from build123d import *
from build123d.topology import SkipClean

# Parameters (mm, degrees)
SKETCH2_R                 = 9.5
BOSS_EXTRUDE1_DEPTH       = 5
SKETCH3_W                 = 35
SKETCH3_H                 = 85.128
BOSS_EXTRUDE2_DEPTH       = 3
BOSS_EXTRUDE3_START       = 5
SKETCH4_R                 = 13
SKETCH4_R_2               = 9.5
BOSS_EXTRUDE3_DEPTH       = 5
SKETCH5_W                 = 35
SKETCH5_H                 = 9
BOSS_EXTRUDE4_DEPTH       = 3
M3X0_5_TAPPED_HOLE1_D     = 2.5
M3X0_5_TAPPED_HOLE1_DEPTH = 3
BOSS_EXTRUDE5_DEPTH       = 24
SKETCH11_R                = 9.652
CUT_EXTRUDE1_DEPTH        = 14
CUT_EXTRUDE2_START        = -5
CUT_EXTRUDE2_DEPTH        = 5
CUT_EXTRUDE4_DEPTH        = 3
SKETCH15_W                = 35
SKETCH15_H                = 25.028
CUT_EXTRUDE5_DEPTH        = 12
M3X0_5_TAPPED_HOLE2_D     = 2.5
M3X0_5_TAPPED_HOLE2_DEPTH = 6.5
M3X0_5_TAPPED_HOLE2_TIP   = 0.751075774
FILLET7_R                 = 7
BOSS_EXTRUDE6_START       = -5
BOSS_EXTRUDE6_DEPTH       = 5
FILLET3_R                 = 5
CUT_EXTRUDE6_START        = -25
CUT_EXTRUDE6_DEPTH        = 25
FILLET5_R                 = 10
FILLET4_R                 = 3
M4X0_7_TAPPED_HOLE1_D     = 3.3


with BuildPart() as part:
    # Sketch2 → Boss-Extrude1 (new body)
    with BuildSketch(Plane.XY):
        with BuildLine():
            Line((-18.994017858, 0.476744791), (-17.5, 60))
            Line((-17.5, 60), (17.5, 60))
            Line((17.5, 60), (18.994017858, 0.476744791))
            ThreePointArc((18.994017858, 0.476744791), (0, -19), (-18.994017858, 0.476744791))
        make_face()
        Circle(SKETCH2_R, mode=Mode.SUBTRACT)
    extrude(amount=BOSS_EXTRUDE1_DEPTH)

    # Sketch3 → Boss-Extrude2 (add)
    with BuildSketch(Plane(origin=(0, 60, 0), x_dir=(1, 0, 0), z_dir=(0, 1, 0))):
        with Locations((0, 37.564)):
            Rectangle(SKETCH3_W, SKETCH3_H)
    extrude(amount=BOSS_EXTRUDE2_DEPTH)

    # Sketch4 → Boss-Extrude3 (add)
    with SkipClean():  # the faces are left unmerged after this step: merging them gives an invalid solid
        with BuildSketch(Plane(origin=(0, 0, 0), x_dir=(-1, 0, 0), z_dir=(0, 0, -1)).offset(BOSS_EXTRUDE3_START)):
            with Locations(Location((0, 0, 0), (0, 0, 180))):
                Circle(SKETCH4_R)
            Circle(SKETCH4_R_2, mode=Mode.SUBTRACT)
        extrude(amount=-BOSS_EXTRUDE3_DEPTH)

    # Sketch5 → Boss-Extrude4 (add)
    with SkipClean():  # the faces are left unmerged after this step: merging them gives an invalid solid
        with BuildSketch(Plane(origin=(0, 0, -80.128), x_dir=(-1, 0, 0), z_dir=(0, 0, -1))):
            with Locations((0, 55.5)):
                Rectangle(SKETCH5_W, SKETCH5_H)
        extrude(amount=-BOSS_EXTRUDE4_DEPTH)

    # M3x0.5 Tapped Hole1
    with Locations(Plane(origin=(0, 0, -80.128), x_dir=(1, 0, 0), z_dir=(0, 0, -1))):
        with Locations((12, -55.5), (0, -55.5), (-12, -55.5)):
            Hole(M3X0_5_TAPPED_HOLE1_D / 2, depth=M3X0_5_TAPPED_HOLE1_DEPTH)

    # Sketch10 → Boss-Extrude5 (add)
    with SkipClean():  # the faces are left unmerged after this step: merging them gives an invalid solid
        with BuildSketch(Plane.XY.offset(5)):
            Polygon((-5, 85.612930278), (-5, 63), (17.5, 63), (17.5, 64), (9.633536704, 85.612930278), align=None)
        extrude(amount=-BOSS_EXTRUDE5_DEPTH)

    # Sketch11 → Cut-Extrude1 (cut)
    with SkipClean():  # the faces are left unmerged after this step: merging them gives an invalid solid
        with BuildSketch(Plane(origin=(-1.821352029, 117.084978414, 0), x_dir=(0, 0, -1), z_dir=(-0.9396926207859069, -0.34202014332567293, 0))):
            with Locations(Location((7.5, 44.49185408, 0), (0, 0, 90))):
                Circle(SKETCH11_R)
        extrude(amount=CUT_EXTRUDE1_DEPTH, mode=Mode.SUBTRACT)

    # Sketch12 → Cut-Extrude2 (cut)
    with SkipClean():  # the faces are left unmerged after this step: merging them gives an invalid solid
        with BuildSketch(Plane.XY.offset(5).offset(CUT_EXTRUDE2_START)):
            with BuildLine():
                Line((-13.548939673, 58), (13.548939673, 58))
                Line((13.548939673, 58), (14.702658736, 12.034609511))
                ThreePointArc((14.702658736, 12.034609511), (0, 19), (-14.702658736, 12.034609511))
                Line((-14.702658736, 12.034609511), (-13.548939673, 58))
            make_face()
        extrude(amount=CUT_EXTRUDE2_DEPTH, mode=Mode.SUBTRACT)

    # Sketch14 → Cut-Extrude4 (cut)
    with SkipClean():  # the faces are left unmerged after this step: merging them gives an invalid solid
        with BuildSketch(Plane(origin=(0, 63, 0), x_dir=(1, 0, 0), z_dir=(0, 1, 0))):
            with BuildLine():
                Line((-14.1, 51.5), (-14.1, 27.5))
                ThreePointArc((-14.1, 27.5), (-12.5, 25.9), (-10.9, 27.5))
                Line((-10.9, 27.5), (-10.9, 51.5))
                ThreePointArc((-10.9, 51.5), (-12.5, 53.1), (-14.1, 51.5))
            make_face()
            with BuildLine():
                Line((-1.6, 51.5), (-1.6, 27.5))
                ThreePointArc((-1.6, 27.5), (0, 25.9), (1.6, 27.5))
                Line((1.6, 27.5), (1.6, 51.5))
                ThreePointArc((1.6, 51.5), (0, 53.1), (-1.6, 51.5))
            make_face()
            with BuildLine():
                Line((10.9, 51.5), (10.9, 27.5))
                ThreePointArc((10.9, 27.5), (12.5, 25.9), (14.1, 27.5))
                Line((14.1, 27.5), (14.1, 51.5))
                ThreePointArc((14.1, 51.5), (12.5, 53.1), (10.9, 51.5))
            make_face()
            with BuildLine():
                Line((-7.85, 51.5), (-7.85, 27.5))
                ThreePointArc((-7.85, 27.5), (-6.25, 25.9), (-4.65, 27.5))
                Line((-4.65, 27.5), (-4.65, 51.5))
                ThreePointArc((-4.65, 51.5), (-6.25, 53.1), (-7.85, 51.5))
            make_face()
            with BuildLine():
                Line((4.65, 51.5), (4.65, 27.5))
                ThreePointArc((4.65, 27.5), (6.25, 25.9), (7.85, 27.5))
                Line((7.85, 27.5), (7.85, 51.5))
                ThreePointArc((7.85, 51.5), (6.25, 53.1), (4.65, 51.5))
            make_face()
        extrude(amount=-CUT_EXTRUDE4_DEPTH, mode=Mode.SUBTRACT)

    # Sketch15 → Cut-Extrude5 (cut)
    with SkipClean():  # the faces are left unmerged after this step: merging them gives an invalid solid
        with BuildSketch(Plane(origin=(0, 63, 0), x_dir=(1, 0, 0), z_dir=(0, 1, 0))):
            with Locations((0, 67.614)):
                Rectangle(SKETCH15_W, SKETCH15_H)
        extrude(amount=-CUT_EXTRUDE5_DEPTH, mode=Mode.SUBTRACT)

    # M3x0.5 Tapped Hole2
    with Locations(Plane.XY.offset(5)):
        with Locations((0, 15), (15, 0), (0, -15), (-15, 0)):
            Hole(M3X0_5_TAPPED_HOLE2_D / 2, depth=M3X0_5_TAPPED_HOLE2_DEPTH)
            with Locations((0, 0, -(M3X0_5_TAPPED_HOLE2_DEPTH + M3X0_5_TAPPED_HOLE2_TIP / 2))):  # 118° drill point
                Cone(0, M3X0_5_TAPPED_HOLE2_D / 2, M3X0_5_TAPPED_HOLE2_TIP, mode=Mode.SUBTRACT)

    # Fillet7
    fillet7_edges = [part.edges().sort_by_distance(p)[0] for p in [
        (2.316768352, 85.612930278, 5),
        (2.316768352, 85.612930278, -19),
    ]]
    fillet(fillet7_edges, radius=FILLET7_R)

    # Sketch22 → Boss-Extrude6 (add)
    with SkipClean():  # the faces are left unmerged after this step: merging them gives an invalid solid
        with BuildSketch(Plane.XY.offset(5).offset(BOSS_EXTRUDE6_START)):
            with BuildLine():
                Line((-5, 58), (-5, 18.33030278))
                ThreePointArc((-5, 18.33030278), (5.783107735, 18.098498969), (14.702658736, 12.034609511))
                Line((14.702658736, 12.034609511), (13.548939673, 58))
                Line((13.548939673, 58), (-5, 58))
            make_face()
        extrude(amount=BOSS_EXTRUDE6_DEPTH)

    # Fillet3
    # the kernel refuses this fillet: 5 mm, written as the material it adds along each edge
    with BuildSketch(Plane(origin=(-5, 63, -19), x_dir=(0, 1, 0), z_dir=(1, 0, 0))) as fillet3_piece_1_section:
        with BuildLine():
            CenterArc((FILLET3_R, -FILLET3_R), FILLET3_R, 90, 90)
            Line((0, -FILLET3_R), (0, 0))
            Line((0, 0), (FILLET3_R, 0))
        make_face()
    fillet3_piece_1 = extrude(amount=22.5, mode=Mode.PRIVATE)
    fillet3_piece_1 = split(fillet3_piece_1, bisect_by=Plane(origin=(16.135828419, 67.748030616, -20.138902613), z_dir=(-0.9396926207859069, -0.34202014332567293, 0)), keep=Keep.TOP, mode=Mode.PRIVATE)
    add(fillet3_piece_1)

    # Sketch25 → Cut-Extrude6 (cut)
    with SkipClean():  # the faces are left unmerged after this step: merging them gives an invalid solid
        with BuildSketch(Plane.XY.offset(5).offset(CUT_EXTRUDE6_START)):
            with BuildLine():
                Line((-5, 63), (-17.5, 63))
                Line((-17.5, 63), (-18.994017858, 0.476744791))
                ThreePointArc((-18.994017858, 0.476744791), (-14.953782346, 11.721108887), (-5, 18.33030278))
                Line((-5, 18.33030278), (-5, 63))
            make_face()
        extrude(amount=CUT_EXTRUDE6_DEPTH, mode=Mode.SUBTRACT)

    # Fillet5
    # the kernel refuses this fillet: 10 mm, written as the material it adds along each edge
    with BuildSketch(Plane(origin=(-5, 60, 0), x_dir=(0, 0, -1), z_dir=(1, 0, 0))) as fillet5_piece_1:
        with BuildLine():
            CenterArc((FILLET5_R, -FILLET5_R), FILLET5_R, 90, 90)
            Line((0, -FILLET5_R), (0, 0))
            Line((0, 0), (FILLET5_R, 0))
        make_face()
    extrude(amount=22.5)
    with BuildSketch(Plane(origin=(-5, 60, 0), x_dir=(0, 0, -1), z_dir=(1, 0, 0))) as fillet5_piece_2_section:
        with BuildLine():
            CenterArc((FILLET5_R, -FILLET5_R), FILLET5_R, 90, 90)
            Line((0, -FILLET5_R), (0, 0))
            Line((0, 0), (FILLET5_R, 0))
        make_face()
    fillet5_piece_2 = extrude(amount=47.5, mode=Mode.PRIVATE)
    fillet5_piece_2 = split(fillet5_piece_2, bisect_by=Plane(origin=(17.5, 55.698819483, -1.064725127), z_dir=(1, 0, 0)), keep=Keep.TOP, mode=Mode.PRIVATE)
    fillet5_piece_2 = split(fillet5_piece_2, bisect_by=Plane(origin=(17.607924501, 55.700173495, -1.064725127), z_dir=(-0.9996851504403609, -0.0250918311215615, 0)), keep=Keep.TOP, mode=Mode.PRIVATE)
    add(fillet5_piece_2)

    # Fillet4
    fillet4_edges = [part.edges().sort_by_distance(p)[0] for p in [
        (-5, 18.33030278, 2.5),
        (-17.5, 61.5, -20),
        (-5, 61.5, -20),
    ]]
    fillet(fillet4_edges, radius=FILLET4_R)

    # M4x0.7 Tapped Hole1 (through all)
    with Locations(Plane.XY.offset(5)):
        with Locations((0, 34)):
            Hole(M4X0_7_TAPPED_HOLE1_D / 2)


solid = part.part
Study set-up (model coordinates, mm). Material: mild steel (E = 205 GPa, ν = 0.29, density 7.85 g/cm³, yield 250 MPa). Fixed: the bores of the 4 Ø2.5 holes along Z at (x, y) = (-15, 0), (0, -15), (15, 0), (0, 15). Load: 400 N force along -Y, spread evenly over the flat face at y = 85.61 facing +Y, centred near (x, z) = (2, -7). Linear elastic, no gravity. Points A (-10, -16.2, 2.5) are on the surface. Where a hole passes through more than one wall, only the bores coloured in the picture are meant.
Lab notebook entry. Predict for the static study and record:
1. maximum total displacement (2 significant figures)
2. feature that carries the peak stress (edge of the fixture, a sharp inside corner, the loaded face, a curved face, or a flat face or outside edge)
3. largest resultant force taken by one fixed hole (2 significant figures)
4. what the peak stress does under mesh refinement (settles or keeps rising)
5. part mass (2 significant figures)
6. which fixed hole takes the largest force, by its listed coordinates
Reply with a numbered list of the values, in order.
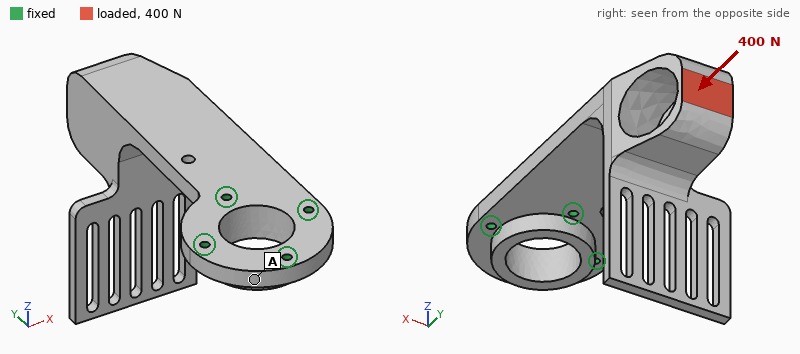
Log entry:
1. 0.22 mm
2. edge of the fixture
3. 290 N
4. keeps rising
5. 160 g
6. (0, 15)
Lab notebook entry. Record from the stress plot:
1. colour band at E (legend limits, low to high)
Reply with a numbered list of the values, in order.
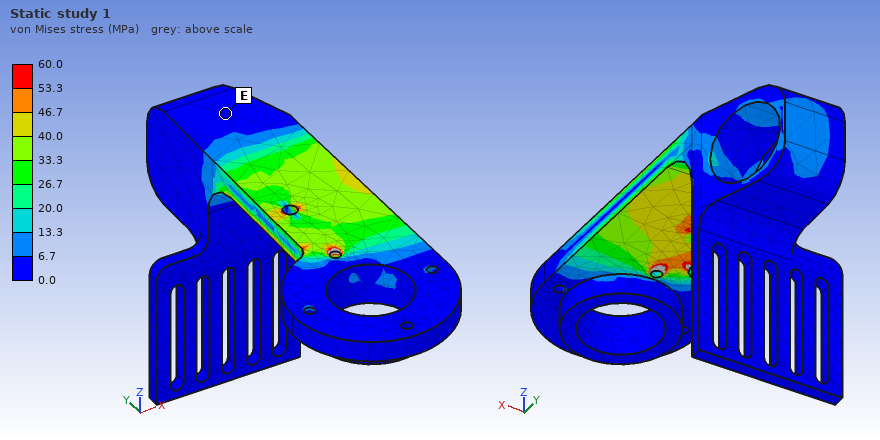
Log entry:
1. 0.0 to 6.7 MPa
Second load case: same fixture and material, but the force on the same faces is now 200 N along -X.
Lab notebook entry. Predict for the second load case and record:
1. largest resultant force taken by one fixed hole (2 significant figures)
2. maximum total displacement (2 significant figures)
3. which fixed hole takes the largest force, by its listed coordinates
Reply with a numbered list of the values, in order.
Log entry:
1. 710 N
2. 85 µm
3. (15, 0)
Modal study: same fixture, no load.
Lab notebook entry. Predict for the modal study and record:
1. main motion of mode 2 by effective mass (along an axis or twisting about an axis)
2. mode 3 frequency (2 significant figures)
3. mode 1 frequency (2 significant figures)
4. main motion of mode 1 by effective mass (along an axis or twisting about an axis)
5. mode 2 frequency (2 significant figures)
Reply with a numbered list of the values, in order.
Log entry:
1. along X
2. 1600 Hz
3. 430 Hz
4. along Z
5. 890 Hz
